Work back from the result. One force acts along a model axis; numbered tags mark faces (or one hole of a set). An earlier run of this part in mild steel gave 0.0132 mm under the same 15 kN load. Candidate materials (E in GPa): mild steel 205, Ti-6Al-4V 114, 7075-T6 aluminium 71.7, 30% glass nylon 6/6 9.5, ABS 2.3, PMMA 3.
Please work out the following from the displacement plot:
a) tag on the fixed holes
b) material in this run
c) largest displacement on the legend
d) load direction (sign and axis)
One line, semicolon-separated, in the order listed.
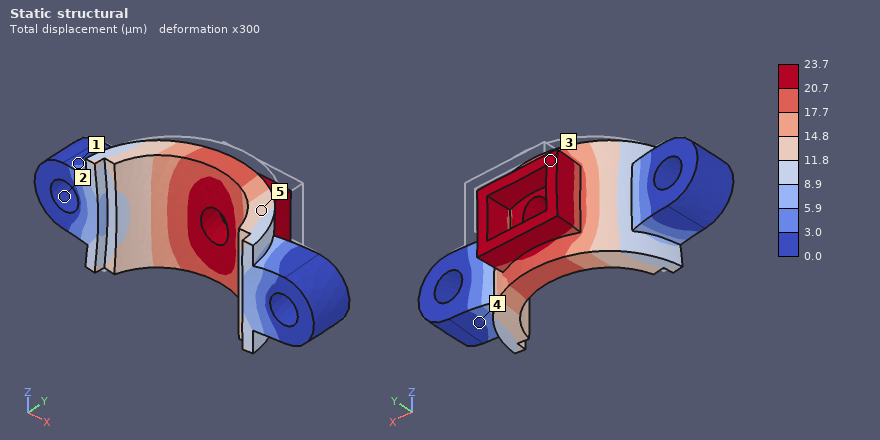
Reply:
2; Ti-6Al-4V; 23.7 µm; -Y
